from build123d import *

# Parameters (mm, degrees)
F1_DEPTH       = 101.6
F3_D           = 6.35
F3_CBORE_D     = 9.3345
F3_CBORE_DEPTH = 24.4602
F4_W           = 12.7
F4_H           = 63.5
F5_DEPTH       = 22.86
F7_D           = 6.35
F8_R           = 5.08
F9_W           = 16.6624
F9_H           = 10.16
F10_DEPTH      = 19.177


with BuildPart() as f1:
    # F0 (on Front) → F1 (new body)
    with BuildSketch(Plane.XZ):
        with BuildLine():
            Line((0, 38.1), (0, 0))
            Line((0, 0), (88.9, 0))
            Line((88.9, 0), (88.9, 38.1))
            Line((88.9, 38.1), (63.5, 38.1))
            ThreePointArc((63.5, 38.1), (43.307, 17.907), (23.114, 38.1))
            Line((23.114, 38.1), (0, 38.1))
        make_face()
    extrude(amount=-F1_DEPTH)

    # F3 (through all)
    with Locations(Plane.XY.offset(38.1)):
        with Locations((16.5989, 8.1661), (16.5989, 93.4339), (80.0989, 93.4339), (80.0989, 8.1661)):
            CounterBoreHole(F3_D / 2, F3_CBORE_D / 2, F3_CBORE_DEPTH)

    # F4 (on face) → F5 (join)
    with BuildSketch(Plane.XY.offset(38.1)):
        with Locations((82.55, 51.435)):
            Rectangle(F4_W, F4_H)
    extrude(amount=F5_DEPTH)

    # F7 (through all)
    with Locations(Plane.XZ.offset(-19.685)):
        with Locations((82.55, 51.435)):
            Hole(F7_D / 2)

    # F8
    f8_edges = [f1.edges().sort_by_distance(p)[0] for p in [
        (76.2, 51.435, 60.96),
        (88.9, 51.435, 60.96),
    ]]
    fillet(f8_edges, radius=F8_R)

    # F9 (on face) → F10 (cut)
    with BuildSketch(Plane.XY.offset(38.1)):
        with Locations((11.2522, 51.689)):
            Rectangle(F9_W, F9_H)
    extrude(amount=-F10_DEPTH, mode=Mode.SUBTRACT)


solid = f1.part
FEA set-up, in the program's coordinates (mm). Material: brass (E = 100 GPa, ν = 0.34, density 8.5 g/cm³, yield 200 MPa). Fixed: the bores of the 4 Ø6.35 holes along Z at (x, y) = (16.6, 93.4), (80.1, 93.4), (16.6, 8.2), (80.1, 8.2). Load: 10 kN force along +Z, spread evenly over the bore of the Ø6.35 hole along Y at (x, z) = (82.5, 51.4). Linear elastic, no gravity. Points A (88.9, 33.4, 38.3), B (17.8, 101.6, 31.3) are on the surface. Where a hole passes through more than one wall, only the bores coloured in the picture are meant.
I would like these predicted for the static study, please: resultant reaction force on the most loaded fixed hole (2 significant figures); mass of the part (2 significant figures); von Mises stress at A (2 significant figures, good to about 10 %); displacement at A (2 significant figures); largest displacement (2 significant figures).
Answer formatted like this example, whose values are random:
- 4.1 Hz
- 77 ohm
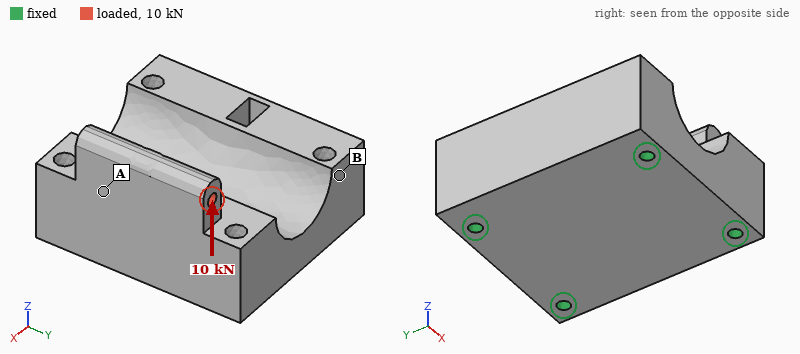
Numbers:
- 5.7 kN
- 2.4 kg
- 12 MPa
- 12 µm
- 17 µm
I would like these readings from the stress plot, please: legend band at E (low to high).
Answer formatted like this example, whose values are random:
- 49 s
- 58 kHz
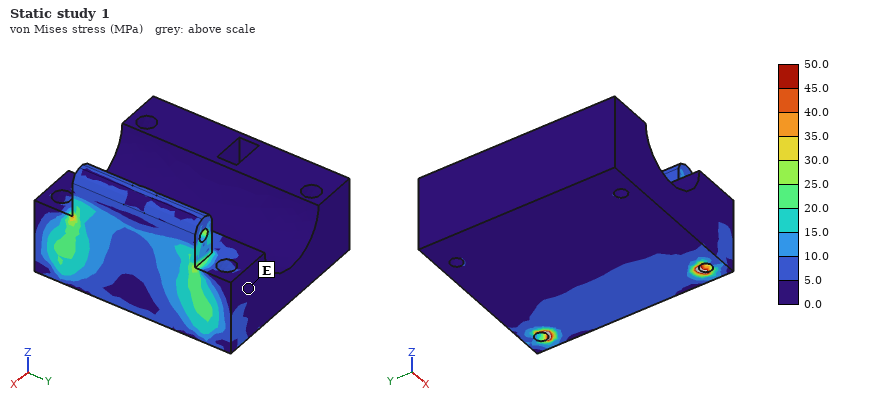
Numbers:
- 0.0 to 5.0 MPa
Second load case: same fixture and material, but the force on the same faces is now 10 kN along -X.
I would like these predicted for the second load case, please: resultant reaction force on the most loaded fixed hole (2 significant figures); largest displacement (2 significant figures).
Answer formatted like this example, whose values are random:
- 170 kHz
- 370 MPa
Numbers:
- 5.1 kN
- 87 µm
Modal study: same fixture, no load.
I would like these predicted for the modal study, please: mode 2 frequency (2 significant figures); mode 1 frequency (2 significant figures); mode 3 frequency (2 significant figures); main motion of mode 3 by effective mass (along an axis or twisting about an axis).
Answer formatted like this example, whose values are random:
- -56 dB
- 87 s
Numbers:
- 5800 Hz
- 4700 Hz
- 6100 Hz
- along Z
